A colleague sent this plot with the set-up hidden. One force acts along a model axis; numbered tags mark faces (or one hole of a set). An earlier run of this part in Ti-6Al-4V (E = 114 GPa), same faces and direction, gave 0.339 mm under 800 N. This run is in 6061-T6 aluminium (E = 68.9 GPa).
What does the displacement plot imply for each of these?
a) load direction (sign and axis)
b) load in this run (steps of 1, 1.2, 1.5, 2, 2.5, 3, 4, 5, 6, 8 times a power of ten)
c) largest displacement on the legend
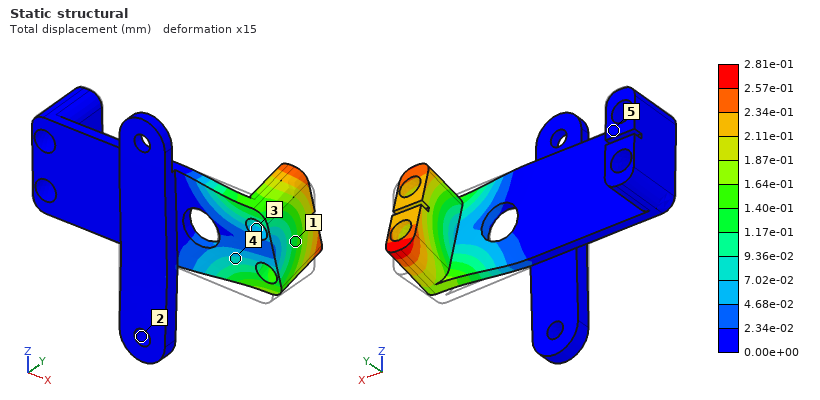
+Z
400 N
2.81e-01 mm
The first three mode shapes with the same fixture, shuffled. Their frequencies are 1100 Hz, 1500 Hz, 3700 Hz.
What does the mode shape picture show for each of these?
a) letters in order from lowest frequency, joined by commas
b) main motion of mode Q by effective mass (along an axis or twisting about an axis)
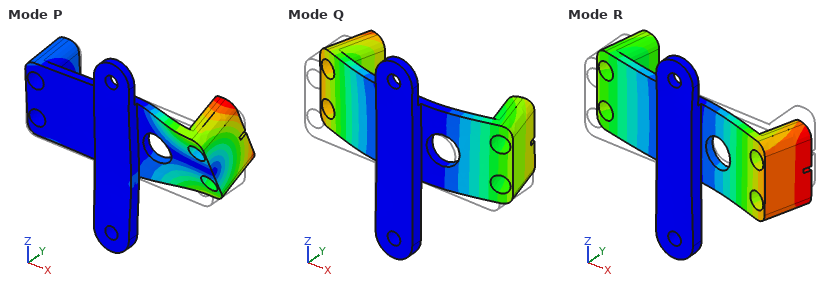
R, Q, P
along Y
